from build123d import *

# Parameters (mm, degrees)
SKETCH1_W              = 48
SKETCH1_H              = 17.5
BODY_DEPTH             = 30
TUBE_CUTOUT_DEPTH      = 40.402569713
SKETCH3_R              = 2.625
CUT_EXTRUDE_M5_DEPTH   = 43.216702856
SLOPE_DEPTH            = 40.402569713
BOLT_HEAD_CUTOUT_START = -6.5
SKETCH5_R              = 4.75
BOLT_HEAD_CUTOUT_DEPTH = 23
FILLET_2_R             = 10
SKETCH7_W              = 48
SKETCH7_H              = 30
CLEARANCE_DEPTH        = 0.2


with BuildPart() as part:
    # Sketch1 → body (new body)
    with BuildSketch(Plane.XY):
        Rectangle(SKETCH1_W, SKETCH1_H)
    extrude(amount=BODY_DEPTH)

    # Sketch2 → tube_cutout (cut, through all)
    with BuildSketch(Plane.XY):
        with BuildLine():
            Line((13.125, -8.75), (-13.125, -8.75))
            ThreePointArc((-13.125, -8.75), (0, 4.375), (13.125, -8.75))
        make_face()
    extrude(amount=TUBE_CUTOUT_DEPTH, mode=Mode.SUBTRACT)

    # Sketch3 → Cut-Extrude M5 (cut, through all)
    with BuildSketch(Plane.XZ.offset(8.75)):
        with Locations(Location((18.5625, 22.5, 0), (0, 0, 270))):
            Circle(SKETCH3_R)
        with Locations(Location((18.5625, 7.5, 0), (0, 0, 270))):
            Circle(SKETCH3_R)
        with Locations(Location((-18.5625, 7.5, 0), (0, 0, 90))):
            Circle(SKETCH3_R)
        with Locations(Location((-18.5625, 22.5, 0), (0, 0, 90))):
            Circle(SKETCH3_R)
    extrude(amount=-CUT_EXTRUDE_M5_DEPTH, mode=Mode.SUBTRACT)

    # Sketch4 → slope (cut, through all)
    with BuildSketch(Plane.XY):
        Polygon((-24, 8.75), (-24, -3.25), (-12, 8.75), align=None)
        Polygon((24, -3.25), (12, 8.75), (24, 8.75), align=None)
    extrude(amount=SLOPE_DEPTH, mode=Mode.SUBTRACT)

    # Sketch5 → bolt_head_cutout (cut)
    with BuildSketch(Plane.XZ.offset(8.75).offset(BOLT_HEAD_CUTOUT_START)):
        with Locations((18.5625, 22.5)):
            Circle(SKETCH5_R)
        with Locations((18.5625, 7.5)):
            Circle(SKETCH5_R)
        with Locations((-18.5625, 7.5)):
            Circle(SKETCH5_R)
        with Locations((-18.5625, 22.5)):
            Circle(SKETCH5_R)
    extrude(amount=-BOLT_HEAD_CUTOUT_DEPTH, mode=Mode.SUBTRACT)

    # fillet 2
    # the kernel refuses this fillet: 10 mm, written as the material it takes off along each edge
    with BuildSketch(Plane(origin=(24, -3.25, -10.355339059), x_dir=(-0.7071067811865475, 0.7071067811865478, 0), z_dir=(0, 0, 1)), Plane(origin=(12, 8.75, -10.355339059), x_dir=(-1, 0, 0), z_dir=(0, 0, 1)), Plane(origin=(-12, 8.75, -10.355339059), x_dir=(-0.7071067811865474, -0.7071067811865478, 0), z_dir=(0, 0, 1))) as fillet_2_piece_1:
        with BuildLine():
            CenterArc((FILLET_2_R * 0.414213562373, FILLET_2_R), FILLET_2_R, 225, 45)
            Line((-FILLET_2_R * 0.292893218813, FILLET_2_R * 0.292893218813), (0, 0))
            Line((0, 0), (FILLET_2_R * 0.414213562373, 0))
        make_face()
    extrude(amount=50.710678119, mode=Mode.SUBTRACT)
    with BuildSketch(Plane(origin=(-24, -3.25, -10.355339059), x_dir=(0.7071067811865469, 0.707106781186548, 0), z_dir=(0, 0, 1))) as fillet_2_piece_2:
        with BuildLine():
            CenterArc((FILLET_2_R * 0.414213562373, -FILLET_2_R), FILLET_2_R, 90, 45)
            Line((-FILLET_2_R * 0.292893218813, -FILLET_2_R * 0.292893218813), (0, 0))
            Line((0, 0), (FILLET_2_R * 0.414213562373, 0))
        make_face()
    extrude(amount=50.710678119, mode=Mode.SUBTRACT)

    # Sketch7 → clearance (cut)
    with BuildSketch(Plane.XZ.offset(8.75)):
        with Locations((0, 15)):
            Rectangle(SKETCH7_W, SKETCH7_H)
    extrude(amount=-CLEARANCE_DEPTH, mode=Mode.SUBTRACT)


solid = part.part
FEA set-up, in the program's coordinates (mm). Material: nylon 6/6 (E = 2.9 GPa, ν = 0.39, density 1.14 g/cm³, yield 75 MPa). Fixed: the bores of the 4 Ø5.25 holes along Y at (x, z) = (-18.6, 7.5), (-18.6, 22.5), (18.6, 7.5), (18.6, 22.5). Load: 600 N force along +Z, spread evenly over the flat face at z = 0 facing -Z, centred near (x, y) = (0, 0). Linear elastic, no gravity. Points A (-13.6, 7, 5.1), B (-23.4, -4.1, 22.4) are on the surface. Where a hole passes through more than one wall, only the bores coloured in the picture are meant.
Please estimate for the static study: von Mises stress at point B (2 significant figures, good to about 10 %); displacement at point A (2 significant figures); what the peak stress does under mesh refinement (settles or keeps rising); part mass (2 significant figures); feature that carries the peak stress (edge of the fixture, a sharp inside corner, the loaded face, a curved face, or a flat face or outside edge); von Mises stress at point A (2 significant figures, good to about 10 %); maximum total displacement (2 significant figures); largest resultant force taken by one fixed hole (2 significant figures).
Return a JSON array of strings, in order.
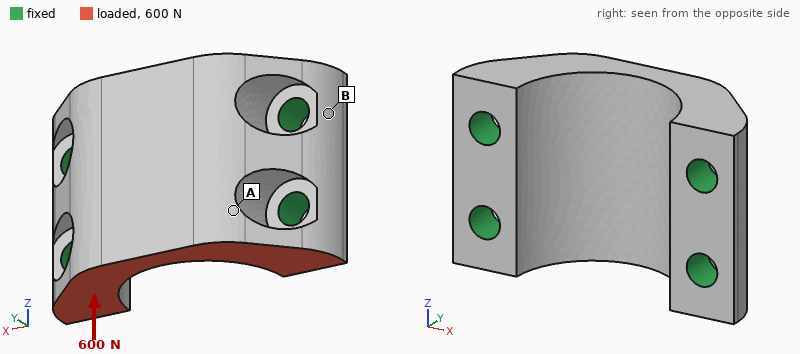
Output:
["0.82 MPa", "29 µm", "keeps rising", "12 g", "edge of the fixture", "2.5 MPa", "39 µm", "230 N"]
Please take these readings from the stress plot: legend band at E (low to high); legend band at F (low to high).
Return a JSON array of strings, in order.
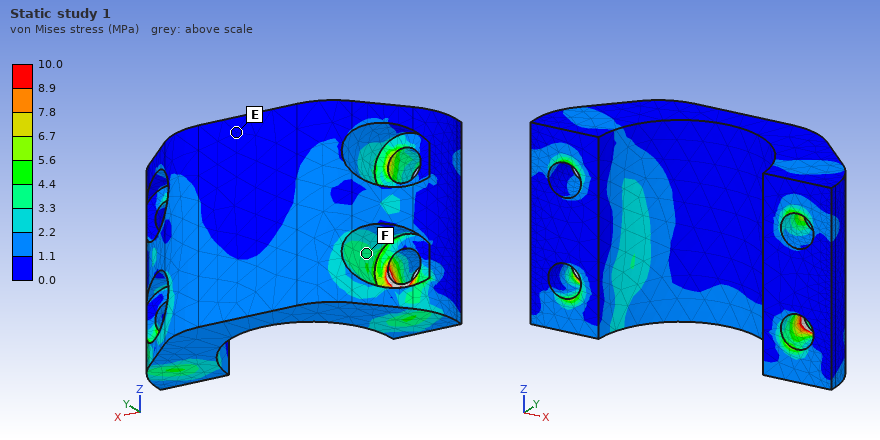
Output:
["0.0 to 1.1 MPa", "3.3 to 4.4 MPa"]
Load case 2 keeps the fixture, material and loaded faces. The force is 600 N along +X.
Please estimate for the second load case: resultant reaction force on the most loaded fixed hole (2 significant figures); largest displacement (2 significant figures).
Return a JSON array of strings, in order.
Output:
["260 N", "70 µm"]
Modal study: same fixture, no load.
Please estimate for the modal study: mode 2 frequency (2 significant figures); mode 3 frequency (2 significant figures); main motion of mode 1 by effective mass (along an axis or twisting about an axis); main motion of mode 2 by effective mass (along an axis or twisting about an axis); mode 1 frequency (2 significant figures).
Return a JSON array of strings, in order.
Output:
["8000 Hz", "9200 Hz", "along Z", "along X", "7100 Hz"]
